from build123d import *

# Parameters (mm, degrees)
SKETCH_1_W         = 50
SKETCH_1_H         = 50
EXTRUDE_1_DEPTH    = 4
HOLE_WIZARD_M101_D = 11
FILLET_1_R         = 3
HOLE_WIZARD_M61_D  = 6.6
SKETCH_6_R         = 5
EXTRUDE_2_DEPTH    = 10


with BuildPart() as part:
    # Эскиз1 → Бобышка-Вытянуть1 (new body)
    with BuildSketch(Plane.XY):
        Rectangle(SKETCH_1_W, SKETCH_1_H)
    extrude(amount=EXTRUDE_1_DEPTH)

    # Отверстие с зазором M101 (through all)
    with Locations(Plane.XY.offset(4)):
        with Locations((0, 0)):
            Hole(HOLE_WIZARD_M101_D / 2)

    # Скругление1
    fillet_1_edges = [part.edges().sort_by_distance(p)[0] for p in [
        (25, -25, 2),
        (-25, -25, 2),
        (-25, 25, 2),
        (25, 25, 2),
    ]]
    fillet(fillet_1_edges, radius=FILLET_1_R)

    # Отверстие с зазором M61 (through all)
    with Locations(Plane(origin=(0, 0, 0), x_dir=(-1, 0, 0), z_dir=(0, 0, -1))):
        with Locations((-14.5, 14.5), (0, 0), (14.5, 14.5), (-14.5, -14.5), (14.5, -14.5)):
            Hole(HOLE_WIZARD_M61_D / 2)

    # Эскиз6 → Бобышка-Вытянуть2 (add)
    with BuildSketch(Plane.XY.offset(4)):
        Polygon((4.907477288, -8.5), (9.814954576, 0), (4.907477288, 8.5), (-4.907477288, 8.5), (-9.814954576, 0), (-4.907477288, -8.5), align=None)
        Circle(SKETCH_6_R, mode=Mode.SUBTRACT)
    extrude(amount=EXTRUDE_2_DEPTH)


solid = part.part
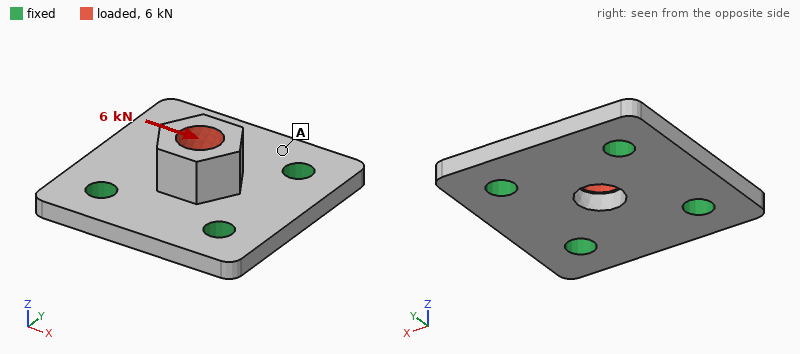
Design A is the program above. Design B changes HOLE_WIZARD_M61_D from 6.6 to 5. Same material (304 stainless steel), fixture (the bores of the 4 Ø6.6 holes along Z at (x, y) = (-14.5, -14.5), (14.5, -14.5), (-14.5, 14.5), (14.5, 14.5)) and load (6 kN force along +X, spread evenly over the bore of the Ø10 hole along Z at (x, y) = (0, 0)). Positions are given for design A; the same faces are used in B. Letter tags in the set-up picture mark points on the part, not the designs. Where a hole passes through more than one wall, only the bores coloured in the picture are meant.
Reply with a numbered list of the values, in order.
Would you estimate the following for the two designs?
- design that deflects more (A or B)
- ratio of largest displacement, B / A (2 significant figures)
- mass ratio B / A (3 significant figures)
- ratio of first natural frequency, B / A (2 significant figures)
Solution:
1. B
2. 1.1
3. 1.02
4. 0.89
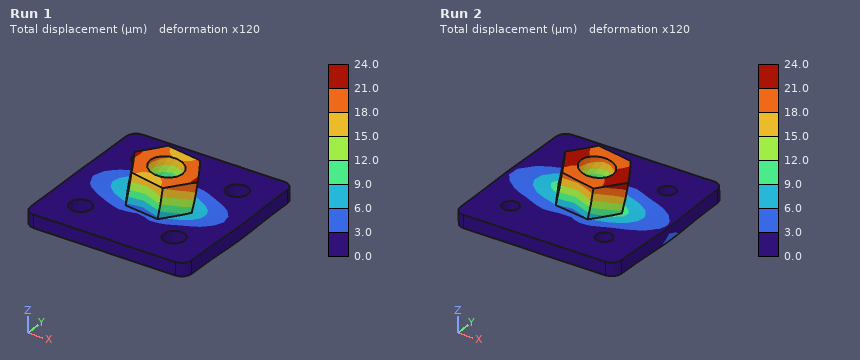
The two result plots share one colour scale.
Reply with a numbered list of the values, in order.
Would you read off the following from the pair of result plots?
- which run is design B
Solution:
1. Run 2
